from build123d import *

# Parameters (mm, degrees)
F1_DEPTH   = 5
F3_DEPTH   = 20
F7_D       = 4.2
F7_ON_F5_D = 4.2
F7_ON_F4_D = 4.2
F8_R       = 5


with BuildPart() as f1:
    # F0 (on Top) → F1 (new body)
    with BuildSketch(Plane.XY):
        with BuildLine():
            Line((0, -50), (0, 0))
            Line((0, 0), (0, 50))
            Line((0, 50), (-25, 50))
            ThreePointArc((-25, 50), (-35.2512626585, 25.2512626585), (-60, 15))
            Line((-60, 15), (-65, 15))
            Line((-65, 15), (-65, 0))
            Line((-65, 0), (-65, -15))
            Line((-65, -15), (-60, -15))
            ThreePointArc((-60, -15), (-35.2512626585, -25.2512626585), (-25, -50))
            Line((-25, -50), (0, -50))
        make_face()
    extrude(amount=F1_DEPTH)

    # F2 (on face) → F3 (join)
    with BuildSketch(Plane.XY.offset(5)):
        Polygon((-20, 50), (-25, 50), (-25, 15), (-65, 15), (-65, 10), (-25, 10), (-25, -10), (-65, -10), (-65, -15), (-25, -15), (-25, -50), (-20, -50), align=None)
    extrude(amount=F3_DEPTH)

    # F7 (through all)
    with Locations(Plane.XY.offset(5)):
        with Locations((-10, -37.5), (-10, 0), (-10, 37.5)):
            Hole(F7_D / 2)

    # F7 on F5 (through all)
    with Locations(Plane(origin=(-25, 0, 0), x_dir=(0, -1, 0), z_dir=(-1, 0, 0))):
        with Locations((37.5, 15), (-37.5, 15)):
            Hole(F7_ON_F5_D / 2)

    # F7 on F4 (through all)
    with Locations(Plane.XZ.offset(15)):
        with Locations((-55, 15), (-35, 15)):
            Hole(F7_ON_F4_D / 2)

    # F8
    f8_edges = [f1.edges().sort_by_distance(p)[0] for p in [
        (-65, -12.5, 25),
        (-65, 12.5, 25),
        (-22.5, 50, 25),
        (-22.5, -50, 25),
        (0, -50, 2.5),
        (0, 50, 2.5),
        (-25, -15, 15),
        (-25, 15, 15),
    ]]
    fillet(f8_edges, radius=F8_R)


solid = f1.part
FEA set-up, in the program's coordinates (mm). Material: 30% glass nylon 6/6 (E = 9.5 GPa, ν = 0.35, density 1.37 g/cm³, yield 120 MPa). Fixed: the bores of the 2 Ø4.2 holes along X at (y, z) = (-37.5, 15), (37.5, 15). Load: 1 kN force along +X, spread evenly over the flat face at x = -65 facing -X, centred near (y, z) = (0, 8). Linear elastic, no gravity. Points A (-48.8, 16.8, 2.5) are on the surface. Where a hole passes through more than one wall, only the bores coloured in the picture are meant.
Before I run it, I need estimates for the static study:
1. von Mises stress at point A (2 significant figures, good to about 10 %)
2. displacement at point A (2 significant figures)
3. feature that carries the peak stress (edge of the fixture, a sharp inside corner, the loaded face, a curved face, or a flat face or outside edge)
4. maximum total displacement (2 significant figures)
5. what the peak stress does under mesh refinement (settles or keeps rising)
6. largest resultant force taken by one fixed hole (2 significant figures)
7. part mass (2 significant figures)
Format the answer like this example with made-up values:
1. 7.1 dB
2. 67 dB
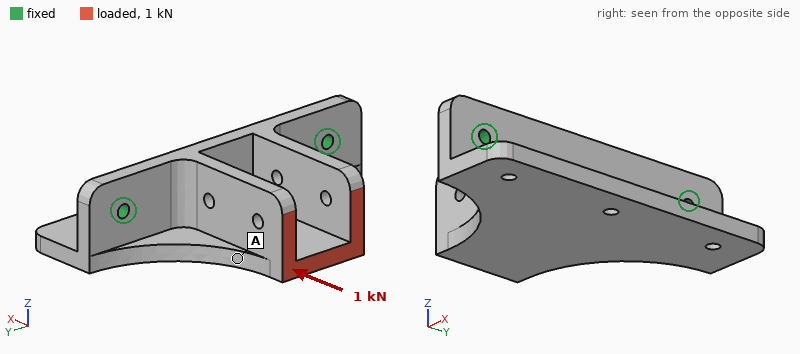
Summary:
1. 5.5 MPa
2. 0.16 mm
3. edge of the fixture
4. 0.22 mm
5. keeps rising
6. 500 N
7. 53 g
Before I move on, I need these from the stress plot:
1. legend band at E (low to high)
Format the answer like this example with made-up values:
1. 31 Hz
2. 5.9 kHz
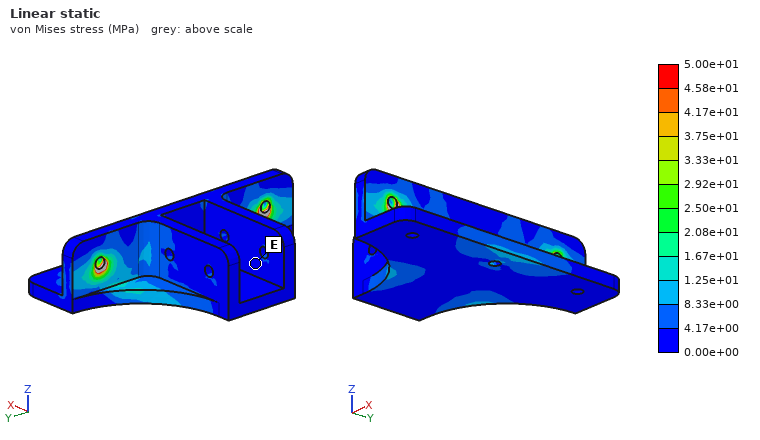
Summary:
1. 0.00e+00 to 4.17e+00 MPa
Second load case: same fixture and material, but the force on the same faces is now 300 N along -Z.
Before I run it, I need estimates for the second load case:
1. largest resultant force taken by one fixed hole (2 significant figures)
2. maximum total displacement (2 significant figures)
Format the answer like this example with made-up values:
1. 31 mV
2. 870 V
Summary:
1. 240 N
2. 1.1 mm
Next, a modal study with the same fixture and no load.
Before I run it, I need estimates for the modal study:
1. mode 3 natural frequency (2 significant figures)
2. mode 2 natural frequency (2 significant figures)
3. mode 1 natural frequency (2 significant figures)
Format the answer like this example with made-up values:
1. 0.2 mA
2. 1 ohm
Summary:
1. 2300 Hz
2. 2300 Hz
3. 880 Hz
